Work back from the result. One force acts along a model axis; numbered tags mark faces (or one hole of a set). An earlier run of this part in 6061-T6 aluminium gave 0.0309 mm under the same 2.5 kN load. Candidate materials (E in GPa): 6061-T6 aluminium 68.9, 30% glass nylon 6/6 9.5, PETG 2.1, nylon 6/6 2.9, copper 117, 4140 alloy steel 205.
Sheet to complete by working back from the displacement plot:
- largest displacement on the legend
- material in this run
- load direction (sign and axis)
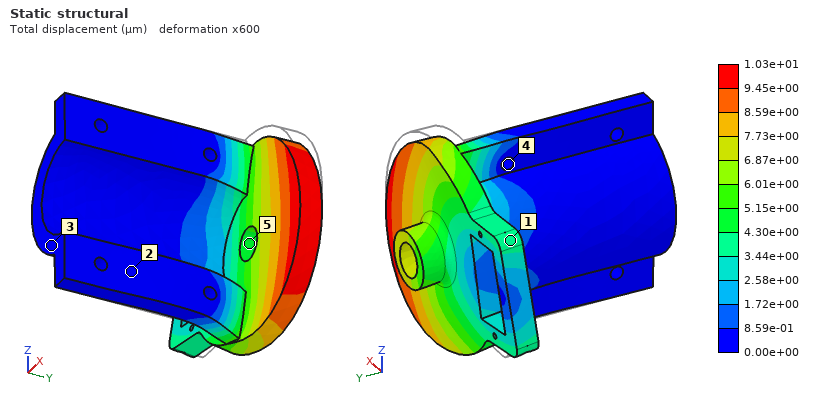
1.03e+01 µm
4140 alloy steel
-Z
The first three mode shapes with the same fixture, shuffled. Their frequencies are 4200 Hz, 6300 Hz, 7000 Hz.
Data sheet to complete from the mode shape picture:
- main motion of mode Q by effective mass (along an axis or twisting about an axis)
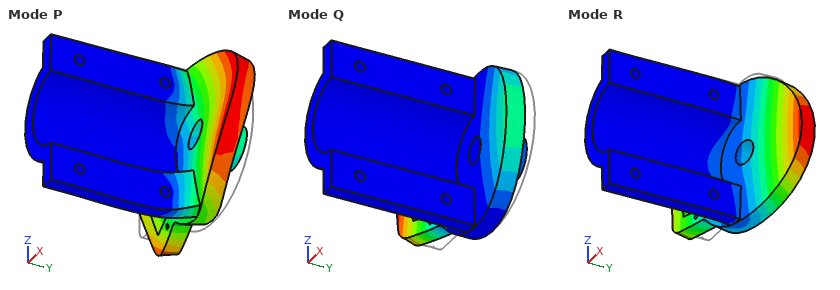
along Y
